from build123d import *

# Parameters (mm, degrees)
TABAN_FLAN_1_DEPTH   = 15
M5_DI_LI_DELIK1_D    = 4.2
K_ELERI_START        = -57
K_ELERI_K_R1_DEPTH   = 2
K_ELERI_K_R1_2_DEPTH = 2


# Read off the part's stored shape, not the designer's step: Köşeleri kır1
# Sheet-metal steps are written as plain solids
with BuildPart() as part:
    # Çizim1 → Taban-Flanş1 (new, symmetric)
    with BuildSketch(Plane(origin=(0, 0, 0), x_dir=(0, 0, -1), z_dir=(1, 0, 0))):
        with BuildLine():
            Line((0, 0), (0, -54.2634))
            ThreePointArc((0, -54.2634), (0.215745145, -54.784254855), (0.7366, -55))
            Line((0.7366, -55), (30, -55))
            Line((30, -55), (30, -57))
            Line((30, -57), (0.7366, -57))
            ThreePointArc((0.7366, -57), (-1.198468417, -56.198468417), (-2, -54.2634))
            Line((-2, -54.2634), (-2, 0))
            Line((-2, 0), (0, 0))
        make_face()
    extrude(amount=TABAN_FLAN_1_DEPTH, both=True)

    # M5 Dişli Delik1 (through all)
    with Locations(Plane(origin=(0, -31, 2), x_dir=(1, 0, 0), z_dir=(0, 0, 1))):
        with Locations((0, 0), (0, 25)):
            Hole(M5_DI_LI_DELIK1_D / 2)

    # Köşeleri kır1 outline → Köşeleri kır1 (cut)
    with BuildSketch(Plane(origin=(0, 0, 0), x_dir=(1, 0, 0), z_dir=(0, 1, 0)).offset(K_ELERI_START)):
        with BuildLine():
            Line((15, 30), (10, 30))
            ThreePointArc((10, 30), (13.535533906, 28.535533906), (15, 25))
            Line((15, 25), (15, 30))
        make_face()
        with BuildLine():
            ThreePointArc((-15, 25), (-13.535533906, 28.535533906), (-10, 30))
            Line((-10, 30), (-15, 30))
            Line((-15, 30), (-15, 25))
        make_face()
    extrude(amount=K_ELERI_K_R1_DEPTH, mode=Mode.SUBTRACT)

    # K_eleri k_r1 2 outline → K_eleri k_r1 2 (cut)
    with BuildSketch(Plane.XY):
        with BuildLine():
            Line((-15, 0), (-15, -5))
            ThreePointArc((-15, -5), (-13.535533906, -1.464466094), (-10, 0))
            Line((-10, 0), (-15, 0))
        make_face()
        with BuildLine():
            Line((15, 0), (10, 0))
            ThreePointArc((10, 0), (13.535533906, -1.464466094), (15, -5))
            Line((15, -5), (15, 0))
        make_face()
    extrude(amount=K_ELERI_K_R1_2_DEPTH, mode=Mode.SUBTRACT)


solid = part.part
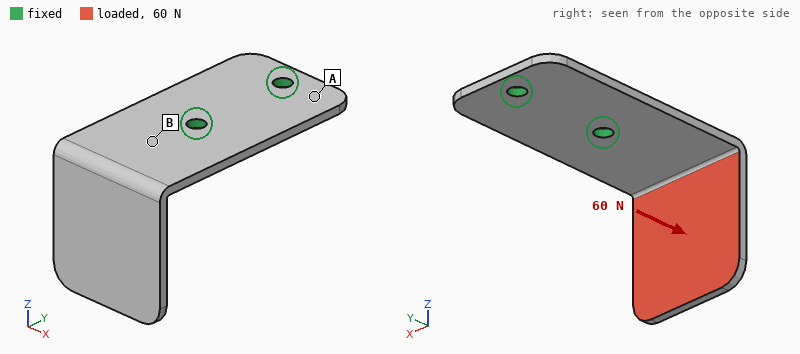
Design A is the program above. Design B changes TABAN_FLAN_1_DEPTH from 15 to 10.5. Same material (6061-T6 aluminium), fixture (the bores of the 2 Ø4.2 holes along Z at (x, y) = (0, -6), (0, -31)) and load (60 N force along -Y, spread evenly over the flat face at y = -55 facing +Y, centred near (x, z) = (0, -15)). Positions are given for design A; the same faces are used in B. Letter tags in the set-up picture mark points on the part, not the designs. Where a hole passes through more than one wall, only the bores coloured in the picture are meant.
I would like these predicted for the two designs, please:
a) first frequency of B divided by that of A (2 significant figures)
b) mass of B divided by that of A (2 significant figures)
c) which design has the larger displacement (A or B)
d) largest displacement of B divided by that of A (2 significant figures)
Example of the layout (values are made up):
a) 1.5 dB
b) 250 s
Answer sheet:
a) 1.0
b) 0.70
c) B
d) 1.4
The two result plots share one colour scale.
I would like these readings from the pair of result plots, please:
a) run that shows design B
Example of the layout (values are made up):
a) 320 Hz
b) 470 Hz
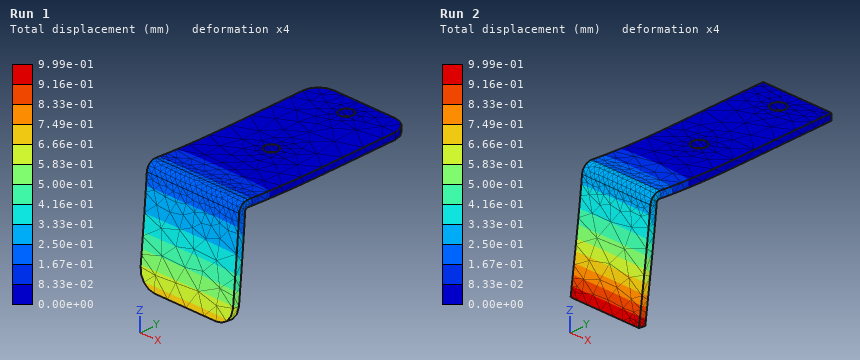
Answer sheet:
a) Run 2
